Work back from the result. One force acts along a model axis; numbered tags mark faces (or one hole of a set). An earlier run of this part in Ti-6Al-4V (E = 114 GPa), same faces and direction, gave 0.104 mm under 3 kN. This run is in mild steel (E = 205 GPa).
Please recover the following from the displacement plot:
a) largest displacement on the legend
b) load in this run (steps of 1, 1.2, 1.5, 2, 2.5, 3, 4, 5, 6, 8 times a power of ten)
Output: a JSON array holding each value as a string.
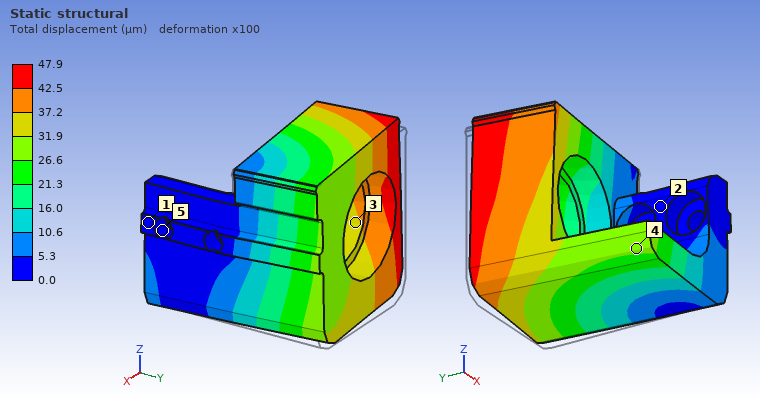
["47.9 µm", "2.5 kN"]
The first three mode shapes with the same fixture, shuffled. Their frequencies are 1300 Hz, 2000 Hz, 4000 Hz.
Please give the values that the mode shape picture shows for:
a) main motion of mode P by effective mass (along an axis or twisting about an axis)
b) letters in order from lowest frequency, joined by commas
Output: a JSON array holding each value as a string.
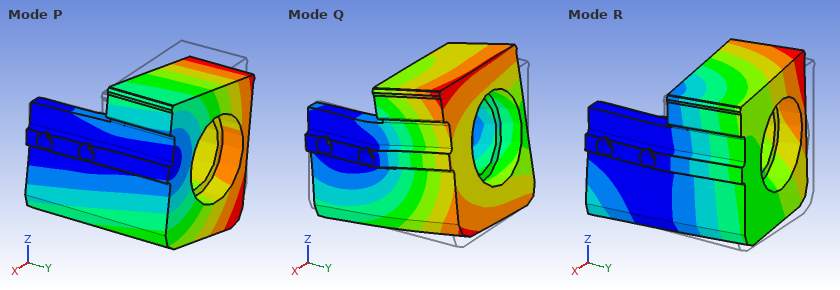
["along Z", "P, R, Q"]
